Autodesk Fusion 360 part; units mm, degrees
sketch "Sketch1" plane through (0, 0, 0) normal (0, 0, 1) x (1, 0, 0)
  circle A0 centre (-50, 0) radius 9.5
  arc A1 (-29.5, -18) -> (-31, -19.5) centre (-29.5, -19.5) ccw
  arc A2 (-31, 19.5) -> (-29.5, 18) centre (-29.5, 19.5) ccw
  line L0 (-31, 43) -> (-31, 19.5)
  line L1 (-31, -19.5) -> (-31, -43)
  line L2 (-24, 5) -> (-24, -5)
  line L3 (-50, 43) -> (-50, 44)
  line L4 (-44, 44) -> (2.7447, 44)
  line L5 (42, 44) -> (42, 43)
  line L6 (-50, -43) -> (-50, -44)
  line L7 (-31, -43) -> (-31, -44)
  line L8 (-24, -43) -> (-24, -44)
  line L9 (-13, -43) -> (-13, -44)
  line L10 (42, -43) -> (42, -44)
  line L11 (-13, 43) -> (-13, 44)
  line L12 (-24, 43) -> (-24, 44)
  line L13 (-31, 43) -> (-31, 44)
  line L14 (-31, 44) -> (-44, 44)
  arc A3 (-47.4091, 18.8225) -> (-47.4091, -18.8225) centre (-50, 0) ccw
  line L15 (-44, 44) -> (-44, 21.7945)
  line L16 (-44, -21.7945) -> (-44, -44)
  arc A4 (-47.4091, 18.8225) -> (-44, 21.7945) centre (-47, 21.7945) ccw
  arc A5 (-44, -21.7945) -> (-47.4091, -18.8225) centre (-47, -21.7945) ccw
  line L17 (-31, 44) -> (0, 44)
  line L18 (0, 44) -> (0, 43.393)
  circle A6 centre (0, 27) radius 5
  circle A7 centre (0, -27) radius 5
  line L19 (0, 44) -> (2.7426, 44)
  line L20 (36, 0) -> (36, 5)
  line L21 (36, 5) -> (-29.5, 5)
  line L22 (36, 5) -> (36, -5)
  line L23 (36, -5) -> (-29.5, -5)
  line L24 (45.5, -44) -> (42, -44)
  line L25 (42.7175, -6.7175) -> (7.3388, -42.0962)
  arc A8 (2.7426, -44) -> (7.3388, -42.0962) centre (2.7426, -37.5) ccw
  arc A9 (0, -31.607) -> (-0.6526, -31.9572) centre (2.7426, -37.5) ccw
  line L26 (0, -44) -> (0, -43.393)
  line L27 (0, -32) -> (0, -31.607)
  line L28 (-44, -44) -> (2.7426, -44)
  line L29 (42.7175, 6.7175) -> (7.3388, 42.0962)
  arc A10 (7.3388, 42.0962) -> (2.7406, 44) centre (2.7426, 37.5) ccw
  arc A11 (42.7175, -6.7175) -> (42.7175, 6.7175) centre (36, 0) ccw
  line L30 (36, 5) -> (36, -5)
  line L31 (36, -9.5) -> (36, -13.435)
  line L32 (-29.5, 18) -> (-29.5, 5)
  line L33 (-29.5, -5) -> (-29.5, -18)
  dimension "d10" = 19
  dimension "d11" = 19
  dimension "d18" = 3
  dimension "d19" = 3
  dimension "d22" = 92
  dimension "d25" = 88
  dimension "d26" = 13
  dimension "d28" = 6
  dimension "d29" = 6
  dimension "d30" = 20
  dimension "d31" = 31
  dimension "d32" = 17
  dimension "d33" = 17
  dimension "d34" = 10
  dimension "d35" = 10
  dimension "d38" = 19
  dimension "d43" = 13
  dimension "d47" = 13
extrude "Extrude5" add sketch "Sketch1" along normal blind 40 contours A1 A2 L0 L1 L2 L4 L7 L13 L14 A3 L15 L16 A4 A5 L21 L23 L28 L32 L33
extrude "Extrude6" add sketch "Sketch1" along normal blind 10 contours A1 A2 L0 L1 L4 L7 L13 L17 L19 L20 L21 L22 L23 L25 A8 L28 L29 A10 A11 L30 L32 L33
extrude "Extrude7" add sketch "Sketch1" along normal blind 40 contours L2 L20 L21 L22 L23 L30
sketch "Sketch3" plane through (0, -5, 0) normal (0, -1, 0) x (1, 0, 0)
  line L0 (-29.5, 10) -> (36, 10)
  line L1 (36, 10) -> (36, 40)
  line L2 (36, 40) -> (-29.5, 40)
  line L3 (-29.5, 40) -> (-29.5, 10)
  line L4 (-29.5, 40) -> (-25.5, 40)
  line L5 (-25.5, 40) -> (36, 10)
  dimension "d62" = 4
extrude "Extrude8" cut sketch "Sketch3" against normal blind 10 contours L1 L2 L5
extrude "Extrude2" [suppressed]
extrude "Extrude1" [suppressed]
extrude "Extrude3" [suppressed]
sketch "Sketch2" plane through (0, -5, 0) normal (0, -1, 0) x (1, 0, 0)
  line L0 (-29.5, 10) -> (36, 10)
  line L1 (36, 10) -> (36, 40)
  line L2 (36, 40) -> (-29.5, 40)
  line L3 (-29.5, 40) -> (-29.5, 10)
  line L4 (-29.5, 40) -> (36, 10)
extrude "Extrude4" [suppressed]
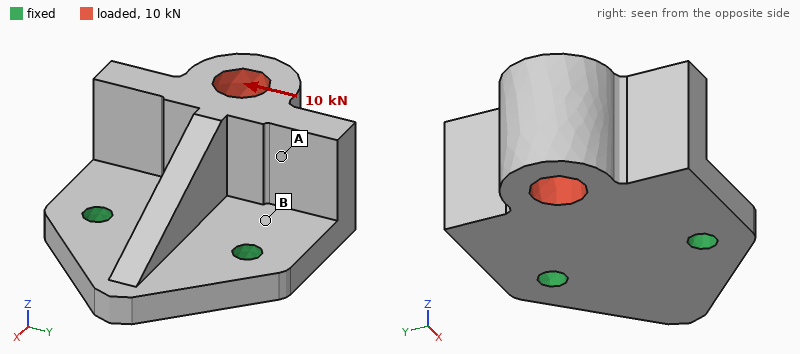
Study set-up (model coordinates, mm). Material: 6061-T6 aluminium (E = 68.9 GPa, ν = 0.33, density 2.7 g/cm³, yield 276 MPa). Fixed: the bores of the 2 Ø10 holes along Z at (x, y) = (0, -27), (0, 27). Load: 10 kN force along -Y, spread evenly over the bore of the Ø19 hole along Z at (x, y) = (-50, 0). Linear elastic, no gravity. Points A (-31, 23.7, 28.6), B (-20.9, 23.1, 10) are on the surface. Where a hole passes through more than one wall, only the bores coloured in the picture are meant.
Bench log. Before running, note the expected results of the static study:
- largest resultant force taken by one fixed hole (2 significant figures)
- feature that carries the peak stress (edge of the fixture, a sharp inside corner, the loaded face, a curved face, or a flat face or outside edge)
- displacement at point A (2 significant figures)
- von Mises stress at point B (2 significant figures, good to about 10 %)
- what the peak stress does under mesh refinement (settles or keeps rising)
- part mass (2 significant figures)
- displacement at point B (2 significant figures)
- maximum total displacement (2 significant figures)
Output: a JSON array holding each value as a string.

["10.0 kN", "edge of the fixture", "66 µm", "50 MPa", "keeps rising", "350 g", "25 µm", "97 µm"]
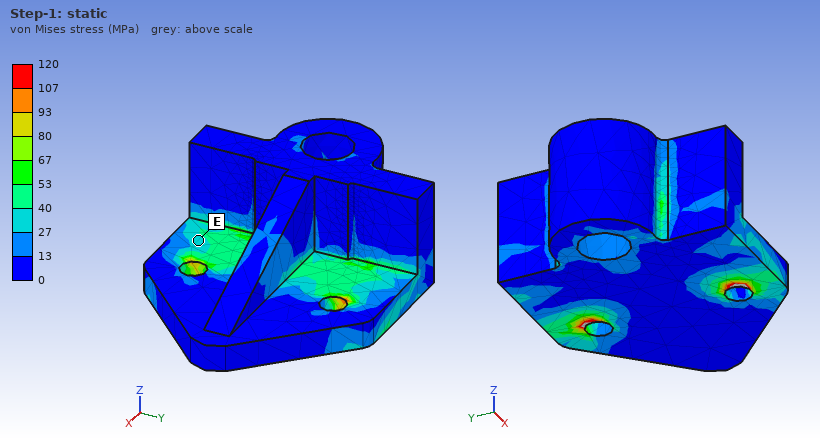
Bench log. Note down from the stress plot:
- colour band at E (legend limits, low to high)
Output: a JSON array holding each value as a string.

["27 to 40 MPa"]
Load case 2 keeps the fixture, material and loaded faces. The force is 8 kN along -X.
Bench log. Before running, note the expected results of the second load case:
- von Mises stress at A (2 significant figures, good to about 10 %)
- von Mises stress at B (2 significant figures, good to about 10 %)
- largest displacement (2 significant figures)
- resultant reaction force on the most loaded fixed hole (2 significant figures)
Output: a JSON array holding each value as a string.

["8.2 MPa", "26 MPa", "0.19 mm", "4.0 kN"]
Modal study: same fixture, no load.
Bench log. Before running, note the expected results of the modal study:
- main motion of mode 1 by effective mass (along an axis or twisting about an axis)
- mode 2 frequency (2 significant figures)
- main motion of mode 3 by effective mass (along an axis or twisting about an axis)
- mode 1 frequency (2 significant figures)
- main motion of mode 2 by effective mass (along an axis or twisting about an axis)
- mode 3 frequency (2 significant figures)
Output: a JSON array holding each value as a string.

["along Z", "3600 Hz", "along Y", "1700 Hz", "along Y", "6500 Hz"]
